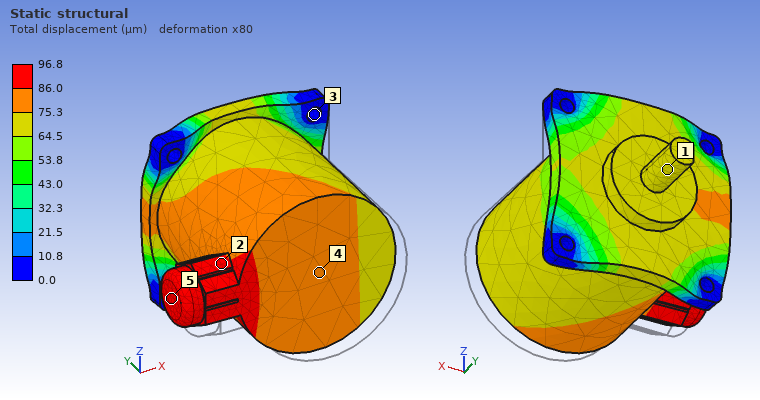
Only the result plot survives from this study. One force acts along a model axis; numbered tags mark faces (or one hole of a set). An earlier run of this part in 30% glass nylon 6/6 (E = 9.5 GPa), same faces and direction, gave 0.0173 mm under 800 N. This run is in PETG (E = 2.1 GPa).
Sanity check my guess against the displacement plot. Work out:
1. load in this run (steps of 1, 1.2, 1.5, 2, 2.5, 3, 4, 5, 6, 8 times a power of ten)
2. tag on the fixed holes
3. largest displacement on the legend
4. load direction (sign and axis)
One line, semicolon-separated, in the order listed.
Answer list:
1 kN; 3; 96.8 µm; +Y
